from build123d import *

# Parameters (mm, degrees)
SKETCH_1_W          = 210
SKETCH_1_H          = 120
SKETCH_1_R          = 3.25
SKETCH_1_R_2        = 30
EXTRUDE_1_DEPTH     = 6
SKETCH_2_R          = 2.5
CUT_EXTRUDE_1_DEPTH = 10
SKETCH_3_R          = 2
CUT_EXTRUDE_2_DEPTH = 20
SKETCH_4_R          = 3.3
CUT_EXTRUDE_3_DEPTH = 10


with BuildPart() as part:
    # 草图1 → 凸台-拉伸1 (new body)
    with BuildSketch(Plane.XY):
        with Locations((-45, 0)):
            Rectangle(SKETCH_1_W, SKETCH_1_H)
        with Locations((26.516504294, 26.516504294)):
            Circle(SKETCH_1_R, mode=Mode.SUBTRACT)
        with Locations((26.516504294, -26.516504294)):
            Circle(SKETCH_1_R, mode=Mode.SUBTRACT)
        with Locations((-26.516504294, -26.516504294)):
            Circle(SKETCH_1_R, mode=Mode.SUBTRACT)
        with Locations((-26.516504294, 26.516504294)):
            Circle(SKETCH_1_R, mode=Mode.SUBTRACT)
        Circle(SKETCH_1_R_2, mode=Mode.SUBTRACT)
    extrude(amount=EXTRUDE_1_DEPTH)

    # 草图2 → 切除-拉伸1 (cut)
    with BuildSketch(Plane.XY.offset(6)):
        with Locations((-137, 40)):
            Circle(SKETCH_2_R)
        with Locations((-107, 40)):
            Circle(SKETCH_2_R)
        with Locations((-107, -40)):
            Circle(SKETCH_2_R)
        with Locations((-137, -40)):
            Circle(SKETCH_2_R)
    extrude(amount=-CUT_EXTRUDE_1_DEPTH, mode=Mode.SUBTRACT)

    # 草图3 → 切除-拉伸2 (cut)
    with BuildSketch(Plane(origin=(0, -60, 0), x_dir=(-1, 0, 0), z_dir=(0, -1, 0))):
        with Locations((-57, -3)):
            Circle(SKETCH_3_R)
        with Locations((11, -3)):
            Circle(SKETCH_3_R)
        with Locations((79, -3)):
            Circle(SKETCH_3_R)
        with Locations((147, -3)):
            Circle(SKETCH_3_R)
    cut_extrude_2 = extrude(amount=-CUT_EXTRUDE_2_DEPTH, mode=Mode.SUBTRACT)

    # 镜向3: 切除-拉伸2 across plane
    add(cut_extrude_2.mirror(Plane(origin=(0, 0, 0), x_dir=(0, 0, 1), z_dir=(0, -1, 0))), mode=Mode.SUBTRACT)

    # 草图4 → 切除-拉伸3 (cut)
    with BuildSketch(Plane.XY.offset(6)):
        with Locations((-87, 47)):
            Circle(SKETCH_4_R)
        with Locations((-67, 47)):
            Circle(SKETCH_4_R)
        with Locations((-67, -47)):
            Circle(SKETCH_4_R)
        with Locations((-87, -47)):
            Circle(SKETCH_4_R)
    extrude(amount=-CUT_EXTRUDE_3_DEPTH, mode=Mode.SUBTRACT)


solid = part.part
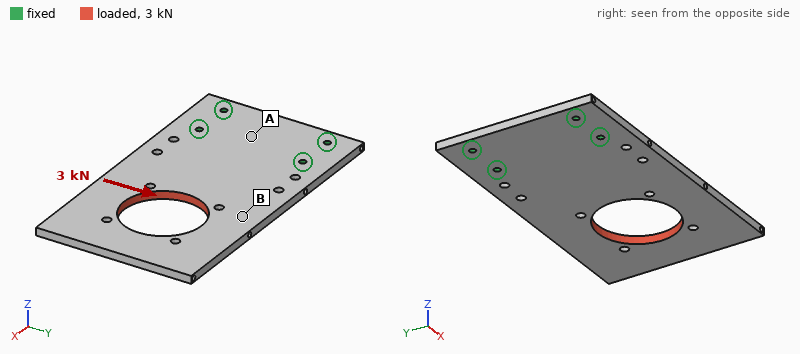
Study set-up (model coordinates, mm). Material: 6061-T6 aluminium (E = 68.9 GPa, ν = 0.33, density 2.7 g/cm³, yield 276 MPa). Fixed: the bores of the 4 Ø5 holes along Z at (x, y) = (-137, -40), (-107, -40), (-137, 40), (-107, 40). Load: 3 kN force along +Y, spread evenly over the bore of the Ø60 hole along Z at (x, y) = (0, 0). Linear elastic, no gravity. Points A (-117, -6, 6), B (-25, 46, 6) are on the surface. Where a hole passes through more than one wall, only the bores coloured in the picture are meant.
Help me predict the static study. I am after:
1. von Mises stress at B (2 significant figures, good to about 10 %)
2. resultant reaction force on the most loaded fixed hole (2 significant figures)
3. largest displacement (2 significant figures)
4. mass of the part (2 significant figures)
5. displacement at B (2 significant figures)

9.5 MPa
3.3 kN
0.11 mm
350 g
0.047 mm
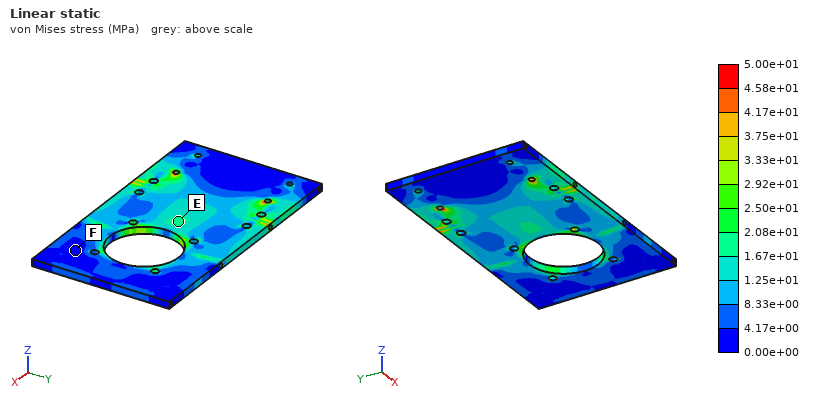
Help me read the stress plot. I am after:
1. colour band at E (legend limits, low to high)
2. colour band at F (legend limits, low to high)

1.67e+01 to 2.08e+01 MPa
0.00e+00 to 4.17e+00 MPa
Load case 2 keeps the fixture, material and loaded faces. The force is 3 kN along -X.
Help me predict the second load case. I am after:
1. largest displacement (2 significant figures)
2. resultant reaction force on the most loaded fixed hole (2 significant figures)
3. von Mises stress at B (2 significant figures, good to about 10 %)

17 µm
1.1 kN
5.1 MPa
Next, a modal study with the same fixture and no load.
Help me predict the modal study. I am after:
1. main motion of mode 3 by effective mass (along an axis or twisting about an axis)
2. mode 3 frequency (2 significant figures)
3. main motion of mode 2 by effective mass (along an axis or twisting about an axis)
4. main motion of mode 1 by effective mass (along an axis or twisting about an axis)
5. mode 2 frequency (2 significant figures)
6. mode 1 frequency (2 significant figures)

along Z
960 Hz
twisting about X
along Z
510 Hz
180 Hz
